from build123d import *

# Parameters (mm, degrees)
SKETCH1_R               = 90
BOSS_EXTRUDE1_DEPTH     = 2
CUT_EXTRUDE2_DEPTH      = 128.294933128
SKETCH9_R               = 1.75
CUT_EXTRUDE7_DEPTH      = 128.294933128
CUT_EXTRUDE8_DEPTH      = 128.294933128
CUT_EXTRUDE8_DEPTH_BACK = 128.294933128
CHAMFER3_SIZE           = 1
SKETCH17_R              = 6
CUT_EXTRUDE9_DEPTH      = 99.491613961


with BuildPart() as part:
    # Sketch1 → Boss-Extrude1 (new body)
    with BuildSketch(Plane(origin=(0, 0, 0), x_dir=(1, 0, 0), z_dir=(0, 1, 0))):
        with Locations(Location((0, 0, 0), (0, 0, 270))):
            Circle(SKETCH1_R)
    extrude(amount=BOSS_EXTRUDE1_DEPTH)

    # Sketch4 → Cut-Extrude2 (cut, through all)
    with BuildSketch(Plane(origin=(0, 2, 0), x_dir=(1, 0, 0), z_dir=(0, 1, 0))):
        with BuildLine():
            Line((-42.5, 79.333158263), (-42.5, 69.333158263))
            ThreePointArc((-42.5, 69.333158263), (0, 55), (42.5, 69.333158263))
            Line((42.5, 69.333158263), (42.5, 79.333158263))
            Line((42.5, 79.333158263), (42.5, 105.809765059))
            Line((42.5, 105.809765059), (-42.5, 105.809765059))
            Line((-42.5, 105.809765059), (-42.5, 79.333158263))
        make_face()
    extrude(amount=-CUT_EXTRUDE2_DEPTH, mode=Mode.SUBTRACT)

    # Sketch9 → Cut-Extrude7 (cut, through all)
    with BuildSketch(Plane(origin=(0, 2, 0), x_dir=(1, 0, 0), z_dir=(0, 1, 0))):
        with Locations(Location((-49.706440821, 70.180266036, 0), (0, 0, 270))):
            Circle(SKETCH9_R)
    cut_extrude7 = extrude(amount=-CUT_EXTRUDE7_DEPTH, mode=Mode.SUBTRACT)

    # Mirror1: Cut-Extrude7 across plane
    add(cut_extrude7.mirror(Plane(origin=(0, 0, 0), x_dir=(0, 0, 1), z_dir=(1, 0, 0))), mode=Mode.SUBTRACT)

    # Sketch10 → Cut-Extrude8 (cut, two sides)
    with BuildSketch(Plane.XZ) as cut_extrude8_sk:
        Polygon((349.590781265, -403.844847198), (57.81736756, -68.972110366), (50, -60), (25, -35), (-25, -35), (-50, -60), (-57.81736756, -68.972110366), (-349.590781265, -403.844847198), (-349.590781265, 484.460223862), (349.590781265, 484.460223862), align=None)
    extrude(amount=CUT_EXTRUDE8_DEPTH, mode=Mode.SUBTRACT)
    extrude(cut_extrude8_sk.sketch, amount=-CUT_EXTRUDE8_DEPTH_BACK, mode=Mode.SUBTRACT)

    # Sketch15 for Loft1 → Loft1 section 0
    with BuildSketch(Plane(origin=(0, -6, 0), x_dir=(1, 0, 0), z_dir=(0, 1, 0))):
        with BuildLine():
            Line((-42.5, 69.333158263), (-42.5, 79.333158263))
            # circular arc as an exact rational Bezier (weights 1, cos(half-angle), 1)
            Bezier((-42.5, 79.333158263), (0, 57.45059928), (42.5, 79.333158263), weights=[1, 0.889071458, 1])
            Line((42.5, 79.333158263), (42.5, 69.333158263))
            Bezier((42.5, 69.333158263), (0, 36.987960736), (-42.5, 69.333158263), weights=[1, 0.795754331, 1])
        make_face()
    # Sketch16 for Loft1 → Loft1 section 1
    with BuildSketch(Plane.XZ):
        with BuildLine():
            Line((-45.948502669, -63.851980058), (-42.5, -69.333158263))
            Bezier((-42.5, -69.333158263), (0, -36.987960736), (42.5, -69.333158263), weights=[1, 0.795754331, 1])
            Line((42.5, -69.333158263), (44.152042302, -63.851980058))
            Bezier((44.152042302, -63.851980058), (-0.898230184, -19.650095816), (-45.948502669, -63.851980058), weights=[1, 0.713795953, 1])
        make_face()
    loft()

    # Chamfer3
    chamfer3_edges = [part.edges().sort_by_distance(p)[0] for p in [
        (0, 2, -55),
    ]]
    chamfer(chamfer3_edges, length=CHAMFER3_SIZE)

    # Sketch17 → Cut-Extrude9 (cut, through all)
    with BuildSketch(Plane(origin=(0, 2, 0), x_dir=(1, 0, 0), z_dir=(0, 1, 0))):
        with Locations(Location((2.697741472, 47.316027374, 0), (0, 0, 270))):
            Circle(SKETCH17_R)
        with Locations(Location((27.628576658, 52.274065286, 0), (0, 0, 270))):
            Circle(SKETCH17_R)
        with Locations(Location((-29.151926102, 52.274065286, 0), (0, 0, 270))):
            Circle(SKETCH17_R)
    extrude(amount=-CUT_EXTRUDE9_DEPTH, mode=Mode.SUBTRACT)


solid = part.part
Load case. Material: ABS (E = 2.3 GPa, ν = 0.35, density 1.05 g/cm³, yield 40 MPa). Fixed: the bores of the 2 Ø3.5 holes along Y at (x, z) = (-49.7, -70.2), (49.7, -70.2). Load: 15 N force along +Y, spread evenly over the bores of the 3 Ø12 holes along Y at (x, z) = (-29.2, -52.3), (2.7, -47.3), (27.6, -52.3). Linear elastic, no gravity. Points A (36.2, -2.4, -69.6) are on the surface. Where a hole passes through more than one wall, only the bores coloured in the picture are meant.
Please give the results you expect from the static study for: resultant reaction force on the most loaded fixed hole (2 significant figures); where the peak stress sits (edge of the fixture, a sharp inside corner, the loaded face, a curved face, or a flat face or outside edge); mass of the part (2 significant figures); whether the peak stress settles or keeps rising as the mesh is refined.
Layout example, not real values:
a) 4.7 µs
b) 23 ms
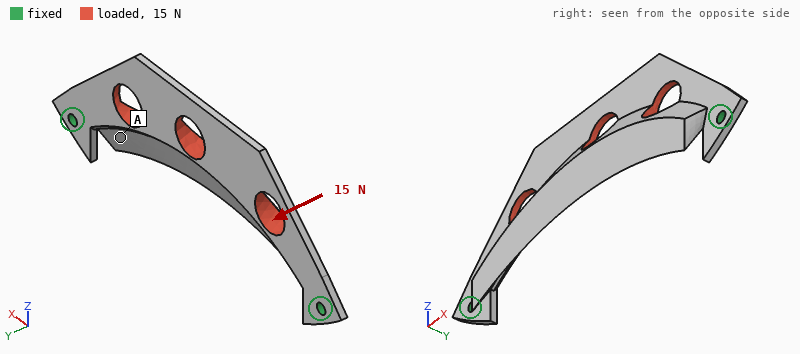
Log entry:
a) 22 N
b) edge of the fixture
c) 9.4 g
d) keeps rising
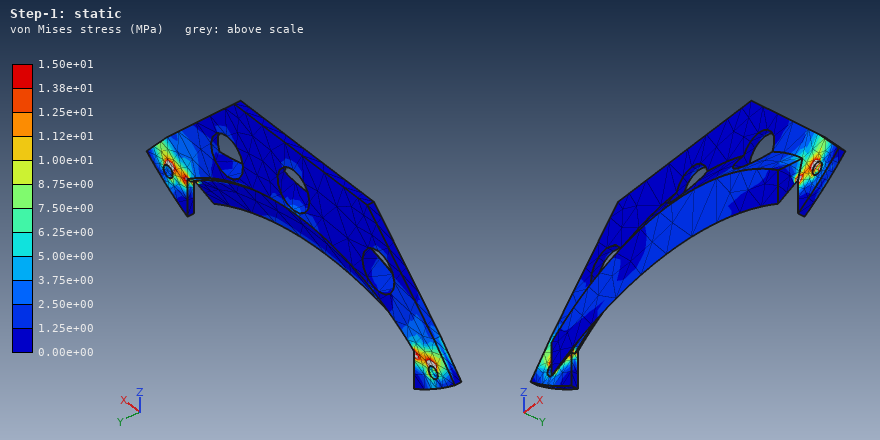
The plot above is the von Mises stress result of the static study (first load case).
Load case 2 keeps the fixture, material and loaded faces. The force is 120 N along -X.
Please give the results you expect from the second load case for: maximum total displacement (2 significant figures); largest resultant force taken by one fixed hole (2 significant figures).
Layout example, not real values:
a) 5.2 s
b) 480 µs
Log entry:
a) 0.18 mm
b) 63 N
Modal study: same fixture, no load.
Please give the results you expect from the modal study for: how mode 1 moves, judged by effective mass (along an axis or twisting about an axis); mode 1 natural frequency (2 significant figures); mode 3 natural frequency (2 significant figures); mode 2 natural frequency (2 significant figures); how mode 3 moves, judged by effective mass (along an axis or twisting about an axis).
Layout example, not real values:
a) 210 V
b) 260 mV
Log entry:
a) along Y
b) 270 Hz
c) 1200 Hz
d) 1000 Hz
e) along Y
